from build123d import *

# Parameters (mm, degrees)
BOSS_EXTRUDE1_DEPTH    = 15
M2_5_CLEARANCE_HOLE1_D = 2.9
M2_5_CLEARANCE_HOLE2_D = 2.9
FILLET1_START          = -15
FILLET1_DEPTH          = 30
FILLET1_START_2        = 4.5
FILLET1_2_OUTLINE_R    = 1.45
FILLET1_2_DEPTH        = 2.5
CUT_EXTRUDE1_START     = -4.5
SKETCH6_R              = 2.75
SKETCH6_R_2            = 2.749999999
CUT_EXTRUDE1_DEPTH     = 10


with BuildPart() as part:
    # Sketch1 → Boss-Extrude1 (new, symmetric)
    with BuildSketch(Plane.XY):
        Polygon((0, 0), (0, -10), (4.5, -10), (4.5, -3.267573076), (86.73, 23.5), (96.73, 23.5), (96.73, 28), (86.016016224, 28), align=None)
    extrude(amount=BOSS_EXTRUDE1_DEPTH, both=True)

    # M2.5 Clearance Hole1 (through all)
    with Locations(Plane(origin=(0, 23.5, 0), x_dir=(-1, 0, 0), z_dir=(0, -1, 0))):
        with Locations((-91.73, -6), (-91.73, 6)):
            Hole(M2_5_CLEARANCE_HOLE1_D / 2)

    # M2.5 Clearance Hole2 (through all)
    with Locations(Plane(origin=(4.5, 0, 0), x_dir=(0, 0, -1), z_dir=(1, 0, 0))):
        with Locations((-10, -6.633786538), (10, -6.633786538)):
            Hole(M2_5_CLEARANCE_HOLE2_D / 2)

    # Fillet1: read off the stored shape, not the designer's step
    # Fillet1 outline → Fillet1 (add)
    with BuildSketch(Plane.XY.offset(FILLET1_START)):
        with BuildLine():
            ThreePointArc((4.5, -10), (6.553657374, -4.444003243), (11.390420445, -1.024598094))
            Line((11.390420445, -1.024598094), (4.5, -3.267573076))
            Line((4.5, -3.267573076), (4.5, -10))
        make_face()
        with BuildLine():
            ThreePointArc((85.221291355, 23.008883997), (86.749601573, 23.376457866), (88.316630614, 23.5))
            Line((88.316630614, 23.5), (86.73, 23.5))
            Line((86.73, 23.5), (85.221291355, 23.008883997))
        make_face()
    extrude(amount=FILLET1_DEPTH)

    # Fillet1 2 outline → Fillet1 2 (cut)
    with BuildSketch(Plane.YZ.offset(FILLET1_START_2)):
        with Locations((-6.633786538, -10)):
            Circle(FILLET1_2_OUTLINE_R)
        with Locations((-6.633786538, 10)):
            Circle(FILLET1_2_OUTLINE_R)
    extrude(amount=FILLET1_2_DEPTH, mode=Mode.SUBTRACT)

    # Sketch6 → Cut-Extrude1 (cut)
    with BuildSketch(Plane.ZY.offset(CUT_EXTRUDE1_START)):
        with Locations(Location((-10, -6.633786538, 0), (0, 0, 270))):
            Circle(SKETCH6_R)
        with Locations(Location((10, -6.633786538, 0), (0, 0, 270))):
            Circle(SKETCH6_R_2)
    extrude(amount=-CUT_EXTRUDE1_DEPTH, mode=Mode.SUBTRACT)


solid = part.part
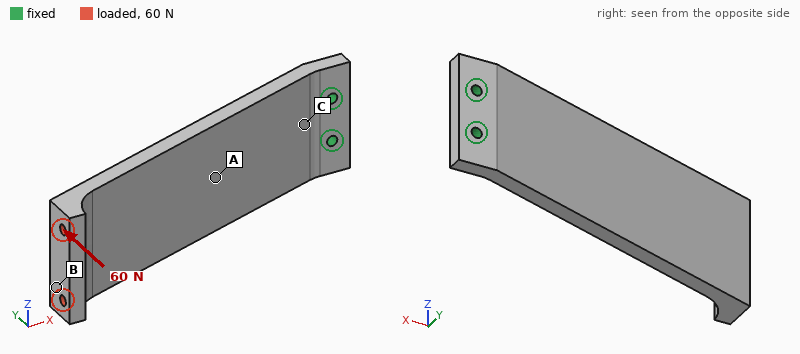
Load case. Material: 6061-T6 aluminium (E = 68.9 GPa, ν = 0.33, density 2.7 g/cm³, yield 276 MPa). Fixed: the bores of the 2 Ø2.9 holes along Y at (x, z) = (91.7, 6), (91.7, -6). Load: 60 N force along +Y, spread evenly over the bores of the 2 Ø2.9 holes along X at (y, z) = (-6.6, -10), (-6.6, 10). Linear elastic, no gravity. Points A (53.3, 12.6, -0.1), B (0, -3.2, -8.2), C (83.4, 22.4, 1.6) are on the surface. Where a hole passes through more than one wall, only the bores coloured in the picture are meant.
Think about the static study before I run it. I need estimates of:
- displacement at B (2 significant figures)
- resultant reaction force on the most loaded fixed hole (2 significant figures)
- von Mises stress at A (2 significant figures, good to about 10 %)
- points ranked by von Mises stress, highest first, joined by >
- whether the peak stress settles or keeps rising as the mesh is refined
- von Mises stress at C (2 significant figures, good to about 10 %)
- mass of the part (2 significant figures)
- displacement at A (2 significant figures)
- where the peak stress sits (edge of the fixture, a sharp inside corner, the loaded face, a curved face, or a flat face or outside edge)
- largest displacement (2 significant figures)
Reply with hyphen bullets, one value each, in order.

- 1.0 mm
- 36 N
- 29 MPa
- C > A > B
- keeps rising
- 46 MPa
- 39 g
- 0.25 mm
- edge of the fixture
- 1.1 mm
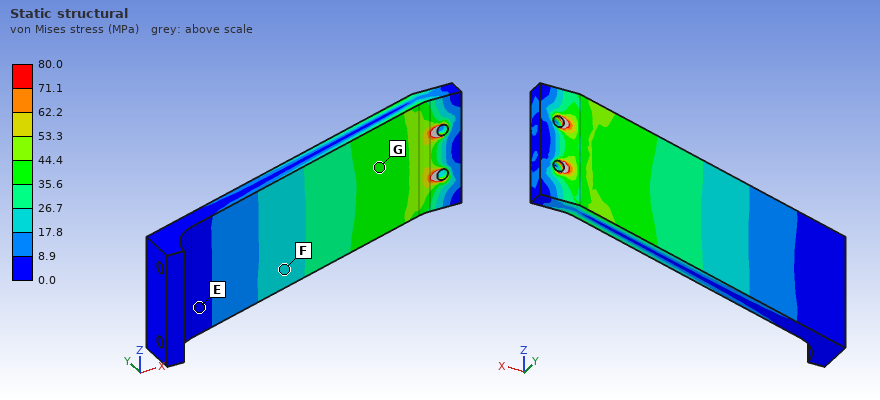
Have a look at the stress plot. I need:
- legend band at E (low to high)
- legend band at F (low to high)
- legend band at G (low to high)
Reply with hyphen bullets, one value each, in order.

- 0.0 to 8.9 MPa
- 17.8 to 26.7 MPa
- 35.6 to 44.4 MPa
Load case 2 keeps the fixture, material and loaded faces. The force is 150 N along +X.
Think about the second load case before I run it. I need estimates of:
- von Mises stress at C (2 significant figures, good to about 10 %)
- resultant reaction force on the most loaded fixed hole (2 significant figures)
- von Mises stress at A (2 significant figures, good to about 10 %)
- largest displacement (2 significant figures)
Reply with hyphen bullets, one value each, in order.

- 46 MPa
- 78 N
- 32 MPa
- 1.1 mm
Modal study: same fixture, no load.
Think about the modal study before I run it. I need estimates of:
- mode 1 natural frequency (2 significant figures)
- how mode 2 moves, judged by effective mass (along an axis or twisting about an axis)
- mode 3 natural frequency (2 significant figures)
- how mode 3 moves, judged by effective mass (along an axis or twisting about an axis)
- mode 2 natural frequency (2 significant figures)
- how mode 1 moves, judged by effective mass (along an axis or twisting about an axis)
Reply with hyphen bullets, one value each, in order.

- 350 Hz
- along Z
- 2200 Hz
- along Y
- 1700 Hz
- along Y
